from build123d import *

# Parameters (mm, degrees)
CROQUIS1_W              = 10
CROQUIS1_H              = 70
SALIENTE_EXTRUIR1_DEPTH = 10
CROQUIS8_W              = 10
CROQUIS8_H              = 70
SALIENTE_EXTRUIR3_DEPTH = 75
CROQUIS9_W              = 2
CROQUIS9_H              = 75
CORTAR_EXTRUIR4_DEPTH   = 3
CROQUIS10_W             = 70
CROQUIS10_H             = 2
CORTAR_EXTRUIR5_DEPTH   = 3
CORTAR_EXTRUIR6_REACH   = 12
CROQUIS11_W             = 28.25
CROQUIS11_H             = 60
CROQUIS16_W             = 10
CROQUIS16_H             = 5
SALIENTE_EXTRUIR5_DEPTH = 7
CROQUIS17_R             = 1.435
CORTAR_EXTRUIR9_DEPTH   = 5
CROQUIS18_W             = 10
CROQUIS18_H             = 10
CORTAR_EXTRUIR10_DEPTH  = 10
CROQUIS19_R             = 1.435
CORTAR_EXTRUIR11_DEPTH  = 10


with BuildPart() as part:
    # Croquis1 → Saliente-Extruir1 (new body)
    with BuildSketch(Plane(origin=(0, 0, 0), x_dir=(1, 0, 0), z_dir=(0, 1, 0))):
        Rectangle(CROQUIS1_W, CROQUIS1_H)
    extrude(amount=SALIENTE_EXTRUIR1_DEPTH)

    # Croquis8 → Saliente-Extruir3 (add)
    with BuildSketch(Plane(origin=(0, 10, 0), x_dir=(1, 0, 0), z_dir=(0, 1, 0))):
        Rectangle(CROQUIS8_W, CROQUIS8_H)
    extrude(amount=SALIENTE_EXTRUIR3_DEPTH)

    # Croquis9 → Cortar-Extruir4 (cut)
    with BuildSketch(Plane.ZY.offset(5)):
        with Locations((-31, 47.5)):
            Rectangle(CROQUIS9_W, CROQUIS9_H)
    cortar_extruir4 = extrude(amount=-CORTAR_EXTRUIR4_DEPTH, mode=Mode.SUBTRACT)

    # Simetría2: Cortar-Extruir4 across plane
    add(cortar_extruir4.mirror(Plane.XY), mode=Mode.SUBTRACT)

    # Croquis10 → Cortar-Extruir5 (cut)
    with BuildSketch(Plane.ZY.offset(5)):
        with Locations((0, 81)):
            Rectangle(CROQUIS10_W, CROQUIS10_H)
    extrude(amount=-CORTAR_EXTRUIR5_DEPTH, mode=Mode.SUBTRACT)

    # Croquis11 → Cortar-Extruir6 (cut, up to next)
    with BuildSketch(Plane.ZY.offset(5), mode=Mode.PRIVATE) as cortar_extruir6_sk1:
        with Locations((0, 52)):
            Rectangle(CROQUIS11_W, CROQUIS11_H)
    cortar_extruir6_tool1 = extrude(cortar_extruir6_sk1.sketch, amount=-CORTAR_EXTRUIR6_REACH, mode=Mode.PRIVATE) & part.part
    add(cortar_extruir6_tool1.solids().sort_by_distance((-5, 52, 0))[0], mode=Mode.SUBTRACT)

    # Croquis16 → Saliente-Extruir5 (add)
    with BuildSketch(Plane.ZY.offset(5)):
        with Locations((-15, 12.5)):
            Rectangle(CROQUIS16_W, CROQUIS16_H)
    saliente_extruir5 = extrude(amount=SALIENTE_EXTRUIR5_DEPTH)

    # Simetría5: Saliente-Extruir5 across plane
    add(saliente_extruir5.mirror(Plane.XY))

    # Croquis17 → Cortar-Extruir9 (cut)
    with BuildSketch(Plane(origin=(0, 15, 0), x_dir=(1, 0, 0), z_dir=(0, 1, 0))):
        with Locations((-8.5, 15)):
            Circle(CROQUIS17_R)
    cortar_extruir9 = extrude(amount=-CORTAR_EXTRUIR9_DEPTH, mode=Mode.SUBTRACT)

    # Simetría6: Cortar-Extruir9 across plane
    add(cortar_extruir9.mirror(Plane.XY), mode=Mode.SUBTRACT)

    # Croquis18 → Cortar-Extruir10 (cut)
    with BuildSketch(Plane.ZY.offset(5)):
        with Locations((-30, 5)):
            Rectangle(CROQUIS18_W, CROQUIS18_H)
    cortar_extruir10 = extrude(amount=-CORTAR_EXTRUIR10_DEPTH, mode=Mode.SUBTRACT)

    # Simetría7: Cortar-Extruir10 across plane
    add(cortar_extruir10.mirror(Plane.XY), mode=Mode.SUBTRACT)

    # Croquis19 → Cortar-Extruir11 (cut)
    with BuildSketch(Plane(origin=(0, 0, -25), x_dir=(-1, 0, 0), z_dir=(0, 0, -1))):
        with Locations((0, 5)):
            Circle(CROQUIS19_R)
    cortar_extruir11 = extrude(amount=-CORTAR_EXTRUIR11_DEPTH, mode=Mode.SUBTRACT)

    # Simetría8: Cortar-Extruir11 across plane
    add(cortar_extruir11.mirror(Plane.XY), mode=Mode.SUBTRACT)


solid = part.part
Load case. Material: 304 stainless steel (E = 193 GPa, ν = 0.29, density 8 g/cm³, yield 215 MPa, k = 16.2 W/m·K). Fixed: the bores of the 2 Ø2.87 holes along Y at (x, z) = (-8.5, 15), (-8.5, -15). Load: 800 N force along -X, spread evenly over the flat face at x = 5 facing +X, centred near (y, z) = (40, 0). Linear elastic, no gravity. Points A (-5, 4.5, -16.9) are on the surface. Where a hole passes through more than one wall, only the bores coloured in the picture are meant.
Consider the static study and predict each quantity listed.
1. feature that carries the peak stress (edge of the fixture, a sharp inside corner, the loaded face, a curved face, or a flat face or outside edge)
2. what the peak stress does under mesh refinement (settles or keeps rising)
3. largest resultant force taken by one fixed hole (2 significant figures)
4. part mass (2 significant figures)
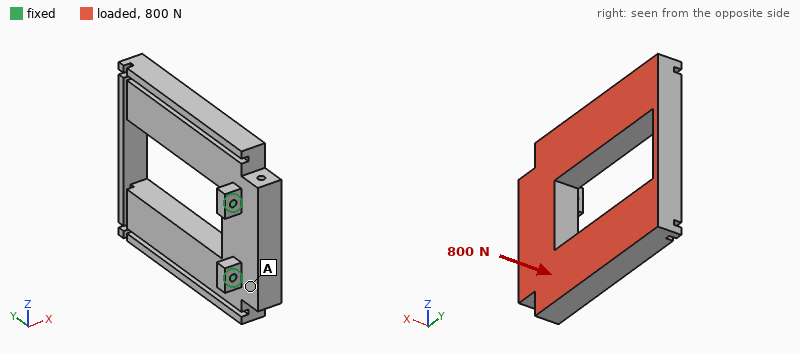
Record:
edge of the fixture
keeps rising
420 N
320 g
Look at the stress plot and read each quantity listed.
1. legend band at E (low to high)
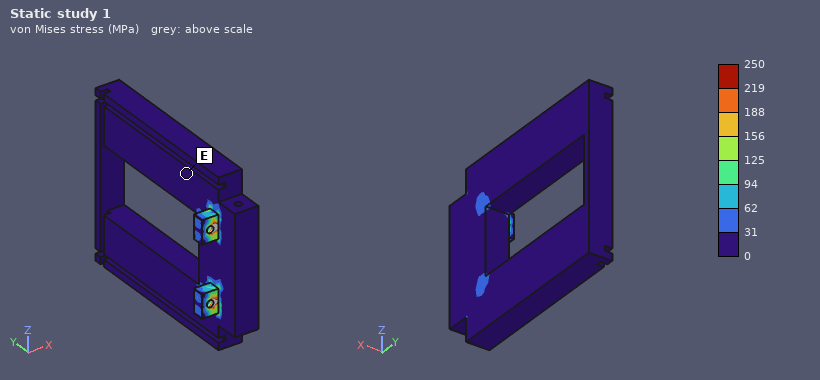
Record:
0 to 31 MPa
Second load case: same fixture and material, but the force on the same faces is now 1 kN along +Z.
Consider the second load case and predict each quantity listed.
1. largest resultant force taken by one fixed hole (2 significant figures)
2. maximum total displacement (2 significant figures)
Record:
1.1 kN
40 µm
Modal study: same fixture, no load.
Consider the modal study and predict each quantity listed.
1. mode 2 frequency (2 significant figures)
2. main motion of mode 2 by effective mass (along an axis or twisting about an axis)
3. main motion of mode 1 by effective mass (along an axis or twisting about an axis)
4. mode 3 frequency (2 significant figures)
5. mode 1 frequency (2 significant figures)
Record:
1700 Hz
along Z
along X
2000 Hz
610 Hz
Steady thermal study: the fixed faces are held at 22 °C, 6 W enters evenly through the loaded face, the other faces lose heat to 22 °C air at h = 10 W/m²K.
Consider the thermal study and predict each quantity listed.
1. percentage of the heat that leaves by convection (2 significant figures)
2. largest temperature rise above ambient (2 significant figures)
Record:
36 %
27 K
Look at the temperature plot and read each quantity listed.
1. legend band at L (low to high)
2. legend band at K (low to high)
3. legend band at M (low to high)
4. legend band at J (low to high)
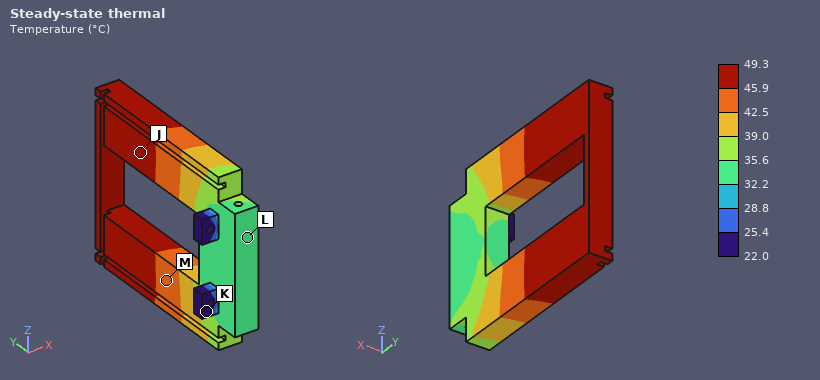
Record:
32.2 to 35.6 °C
22.0 to 25.4 °C
42.5 to 45.9 °C
45.9 to 49.3 °C
